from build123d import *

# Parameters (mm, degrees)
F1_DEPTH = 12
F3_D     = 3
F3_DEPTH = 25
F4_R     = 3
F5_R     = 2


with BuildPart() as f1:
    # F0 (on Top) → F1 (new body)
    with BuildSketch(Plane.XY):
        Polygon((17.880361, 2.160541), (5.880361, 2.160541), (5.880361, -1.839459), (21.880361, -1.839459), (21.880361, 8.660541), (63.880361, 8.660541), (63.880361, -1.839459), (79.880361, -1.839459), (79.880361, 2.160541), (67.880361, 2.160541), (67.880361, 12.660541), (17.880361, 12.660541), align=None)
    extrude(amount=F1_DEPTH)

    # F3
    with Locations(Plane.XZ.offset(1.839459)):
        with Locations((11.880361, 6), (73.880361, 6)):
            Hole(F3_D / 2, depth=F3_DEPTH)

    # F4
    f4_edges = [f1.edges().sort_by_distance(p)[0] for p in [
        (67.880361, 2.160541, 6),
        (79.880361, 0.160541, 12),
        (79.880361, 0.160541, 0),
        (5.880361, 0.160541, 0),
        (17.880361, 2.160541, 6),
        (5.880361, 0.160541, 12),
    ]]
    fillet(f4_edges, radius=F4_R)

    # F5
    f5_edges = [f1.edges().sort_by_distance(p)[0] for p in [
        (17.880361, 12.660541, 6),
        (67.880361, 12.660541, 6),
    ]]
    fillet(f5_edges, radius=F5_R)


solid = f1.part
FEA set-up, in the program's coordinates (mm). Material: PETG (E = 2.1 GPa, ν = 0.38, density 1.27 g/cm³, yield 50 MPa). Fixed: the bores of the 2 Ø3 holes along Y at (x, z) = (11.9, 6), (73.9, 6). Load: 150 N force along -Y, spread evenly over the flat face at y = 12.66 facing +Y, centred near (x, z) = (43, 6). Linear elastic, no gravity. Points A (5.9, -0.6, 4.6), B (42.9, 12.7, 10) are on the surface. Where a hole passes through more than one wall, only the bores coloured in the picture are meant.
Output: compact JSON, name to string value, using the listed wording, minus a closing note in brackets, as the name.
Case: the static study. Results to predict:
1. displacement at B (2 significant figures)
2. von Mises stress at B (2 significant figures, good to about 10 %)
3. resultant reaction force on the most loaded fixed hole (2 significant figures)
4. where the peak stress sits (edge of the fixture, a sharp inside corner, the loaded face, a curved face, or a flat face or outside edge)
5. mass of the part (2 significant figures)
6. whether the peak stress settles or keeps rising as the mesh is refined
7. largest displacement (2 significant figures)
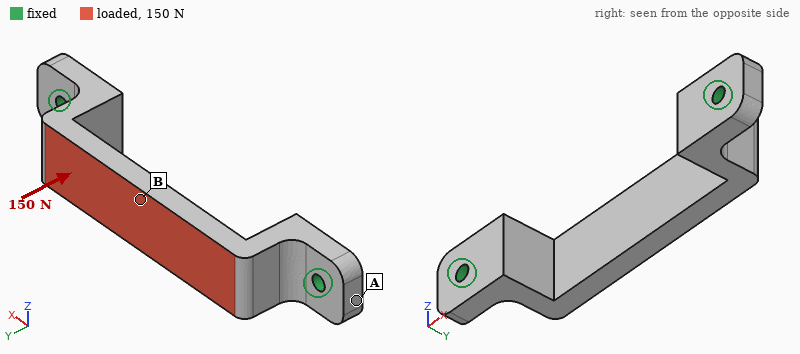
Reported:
{"displacement at B": "0.40 mm", "von Mises stress at B": "12 MPa", "resultant reaction force on the most loaded fixed hole": "110 N", "where the peak stress sits": "edge of the fixture", "mass of the part": "5.7 g", "whether the peak stress settles or keeps rising as the mesh is refined": "keeps rising", "largest displacement": "0.41 mm"}
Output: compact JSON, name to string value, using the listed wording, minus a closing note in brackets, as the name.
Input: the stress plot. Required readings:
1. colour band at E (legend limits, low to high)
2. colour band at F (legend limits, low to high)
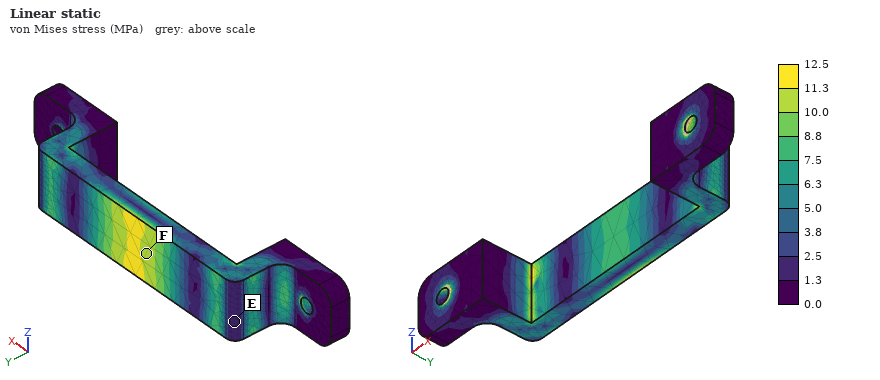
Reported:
{"colour band at E": "1.3 to 2.5 MPa", "colour band at F": "10.0 to 11.3 MPa"}
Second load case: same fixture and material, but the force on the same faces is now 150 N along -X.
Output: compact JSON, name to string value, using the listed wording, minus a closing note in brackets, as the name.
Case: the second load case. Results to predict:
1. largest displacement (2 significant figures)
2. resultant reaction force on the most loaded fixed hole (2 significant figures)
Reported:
{"largest displacement": "0.23 mm", "resultant reaction force on the most loaded fixed hole": "78 N"}
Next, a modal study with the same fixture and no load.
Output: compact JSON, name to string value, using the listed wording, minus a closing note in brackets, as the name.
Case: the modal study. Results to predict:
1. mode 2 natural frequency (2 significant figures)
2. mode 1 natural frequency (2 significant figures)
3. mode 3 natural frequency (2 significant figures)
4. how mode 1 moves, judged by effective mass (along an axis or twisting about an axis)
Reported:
{"mode 2 natural frequency": "2100 Hz", "mode 1 natural frequency": "1600 Hz", "mode 3 natural frequency": "2100 Hz", "how mode 1 moves, judged by effective mass": "along Z"}
